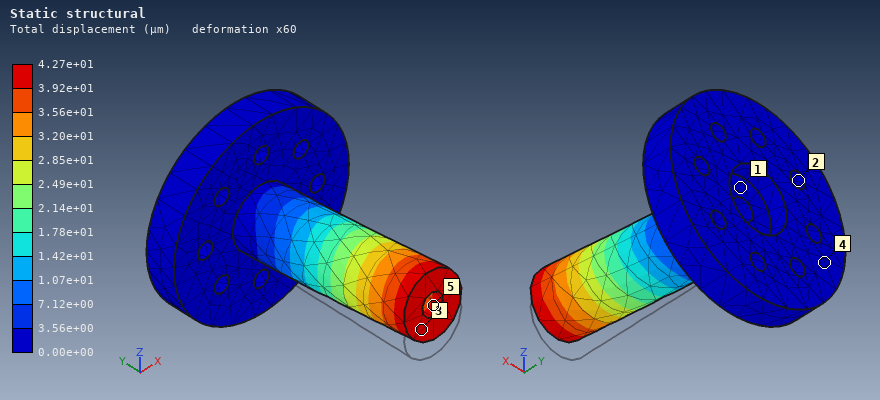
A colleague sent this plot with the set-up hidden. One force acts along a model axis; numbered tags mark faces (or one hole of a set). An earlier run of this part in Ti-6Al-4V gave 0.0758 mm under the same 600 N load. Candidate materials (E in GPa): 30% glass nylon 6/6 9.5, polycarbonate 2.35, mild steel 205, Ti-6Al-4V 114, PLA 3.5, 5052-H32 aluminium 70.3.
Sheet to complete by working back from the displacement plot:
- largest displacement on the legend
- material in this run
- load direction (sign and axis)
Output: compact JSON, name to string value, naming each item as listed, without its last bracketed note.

{"largest displacement on the legend": "4.27e+01 µm", "material in this run": "mild steel", "load direction": "+Z"}
